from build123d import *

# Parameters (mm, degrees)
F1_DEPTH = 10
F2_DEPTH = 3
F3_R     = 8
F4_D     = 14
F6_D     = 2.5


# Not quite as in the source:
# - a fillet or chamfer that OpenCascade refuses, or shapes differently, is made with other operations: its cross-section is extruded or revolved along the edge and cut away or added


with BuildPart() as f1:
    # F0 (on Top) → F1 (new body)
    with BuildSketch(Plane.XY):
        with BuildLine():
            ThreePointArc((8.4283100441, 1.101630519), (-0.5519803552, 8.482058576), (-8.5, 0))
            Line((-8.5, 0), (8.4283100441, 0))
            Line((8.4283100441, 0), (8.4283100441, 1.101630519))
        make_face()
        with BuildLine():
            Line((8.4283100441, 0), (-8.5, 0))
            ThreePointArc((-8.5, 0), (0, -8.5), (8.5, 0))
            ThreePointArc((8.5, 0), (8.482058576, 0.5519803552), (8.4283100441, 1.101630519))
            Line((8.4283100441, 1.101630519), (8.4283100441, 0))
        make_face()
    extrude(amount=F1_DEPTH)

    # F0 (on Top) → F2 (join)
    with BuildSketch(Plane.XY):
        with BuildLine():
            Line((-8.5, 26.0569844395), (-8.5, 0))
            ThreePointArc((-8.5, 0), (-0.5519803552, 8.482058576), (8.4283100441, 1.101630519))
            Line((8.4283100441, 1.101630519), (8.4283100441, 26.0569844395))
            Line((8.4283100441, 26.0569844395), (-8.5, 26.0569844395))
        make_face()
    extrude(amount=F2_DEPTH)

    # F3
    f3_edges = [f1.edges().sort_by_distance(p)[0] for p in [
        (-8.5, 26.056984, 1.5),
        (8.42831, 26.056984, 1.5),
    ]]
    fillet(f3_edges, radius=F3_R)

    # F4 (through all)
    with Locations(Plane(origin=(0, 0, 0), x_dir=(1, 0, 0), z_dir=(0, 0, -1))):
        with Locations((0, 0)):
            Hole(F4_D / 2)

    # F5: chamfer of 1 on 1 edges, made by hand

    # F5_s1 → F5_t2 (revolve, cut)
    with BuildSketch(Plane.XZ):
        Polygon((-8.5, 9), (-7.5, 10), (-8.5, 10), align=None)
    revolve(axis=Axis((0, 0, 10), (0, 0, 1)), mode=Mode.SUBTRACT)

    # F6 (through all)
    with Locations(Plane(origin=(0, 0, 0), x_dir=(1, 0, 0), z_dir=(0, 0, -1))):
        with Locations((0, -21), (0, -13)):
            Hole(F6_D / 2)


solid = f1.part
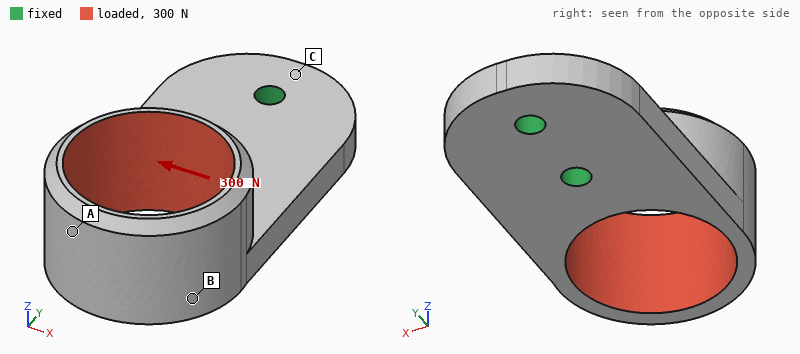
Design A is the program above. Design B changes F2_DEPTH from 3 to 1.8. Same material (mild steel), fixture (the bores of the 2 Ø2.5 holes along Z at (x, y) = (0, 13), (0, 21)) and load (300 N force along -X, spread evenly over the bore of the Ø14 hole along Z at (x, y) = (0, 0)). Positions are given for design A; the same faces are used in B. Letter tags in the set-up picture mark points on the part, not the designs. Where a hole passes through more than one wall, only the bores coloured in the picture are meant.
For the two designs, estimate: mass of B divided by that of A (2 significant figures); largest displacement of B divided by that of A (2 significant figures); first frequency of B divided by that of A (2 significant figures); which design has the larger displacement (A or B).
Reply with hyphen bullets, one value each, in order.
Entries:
- 0.78
- 1.9
- 0.54
- B
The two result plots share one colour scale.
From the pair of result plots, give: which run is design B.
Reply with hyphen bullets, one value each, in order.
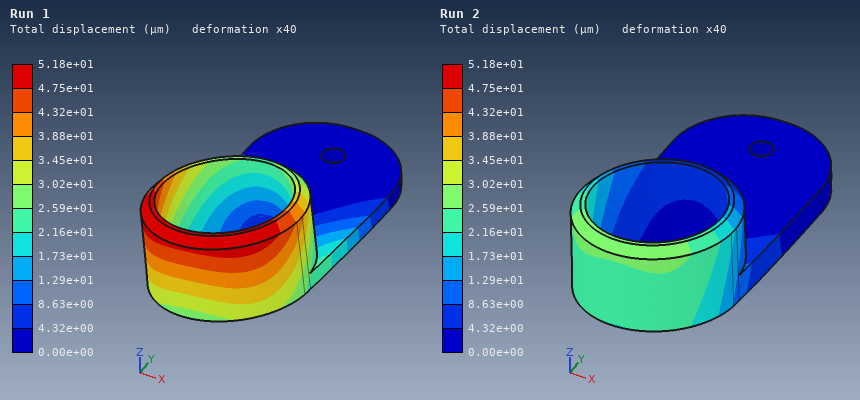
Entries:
- Run 1
